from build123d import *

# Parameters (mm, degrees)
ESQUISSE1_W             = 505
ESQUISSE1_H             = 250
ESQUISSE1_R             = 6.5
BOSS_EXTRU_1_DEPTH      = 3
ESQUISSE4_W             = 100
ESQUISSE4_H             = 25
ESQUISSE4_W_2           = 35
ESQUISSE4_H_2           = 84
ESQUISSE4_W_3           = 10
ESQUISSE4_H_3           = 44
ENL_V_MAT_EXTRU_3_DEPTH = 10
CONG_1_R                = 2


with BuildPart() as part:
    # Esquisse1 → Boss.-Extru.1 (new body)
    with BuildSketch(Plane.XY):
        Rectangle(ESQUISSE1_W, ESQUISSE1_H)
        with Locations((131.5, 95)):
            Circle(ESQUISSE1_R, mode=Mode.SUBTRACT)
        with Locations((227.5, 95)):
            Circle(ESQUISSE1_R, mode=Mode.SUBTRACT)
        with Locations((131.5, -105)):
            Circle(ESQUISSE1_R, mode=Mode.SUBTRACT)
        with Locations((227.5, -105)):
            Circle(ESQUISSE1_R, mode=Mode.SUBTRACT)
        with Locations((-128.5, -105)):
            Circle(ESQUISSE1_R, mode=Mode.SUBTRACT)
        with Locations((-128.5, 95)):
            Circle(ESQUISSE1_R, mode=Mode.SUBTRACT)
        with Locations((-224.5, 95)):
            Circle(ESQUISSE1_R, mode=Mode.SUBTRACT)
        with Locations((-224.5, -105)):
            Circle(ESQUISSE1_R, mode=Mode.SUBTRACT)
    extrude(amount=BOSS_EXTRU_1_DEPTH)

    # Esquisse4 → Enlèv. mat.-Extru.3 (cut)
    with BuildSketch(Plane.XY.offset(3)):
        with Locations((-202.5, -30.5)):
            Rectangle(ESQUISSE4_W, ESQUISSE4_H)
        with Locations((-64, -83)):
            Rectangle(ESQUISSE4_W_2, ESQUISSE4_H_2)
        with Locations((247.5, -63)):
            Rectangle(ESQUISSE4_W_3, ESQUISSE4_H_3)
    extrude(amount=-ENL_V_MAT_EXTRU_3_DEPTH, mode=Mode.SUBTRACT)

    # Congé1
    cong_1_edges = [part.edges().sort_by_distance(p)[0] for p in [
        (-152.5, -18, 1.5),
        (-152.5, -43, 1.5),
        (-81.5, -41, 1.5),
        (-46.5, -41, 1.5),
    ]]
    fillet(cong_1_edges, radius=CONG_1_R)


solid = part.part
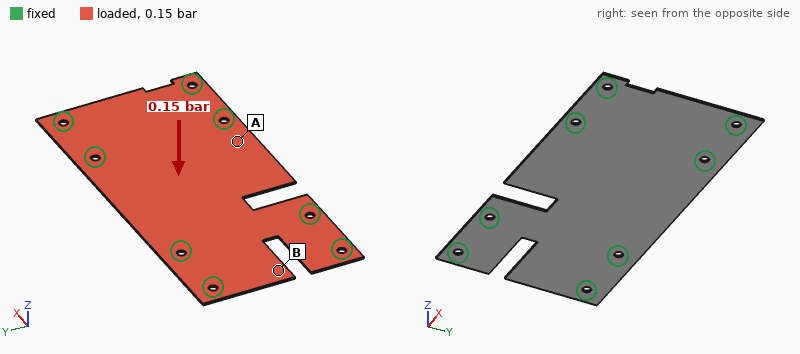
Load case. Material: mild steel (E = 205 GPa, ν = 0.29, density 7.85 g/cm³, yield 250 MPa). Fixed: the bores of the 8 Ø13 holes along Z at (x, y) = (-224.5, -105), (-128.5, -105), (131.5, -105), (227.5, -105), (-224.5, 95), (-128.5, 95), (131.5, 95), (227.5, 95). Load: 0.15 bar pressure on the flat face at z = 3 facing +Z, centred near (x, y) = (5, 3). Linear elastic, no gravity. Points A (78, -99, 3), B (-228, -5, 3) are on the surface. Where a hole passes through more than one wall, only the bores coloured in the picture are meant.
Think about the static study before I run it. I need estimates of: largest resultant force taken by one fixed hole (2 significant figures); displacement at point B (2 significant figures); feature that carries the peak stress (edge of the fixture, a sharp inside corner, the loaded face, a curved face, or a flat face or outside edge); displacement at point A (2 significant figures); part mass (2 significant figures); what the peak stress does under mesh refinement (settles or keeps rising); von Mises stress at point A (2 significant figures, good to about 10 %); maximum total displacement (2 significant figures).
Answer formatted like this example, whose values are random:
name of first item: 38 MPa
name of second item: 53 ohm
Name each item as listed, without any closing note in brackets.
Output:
largest resultant force taken by one fixed hole: 370 N
displacement at point B: 0.24 mm
feature that carries the peak stress: edge of the fixture
displacement at point A: 0.27 mm
part mass: 2.8 kg
what the peak stress does under mesh refinement: keeps rising
von Mises stress at point A: 15 MPa
maximum total displacement: 1.0 mm
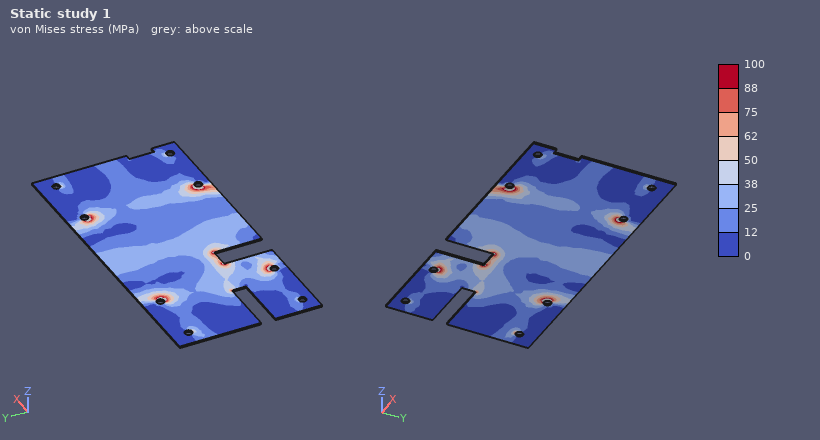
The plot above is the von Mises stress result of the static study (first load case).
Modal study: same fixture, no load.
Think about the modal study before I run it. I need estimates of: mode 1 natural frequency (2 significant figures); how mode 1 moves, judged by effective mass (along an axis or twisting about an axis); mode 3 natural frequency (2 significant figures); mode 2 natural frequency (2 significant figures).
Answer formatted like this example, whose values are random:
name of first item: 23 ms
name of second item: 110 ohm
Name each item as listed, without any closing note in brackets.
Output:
mode 1 natural frequency: 170 Hz
how mode 1 moves, judged by effective mass: along Z
mode 3 natural frequency: 320 Hz
mode 2 natural frequency: 250 Hz
